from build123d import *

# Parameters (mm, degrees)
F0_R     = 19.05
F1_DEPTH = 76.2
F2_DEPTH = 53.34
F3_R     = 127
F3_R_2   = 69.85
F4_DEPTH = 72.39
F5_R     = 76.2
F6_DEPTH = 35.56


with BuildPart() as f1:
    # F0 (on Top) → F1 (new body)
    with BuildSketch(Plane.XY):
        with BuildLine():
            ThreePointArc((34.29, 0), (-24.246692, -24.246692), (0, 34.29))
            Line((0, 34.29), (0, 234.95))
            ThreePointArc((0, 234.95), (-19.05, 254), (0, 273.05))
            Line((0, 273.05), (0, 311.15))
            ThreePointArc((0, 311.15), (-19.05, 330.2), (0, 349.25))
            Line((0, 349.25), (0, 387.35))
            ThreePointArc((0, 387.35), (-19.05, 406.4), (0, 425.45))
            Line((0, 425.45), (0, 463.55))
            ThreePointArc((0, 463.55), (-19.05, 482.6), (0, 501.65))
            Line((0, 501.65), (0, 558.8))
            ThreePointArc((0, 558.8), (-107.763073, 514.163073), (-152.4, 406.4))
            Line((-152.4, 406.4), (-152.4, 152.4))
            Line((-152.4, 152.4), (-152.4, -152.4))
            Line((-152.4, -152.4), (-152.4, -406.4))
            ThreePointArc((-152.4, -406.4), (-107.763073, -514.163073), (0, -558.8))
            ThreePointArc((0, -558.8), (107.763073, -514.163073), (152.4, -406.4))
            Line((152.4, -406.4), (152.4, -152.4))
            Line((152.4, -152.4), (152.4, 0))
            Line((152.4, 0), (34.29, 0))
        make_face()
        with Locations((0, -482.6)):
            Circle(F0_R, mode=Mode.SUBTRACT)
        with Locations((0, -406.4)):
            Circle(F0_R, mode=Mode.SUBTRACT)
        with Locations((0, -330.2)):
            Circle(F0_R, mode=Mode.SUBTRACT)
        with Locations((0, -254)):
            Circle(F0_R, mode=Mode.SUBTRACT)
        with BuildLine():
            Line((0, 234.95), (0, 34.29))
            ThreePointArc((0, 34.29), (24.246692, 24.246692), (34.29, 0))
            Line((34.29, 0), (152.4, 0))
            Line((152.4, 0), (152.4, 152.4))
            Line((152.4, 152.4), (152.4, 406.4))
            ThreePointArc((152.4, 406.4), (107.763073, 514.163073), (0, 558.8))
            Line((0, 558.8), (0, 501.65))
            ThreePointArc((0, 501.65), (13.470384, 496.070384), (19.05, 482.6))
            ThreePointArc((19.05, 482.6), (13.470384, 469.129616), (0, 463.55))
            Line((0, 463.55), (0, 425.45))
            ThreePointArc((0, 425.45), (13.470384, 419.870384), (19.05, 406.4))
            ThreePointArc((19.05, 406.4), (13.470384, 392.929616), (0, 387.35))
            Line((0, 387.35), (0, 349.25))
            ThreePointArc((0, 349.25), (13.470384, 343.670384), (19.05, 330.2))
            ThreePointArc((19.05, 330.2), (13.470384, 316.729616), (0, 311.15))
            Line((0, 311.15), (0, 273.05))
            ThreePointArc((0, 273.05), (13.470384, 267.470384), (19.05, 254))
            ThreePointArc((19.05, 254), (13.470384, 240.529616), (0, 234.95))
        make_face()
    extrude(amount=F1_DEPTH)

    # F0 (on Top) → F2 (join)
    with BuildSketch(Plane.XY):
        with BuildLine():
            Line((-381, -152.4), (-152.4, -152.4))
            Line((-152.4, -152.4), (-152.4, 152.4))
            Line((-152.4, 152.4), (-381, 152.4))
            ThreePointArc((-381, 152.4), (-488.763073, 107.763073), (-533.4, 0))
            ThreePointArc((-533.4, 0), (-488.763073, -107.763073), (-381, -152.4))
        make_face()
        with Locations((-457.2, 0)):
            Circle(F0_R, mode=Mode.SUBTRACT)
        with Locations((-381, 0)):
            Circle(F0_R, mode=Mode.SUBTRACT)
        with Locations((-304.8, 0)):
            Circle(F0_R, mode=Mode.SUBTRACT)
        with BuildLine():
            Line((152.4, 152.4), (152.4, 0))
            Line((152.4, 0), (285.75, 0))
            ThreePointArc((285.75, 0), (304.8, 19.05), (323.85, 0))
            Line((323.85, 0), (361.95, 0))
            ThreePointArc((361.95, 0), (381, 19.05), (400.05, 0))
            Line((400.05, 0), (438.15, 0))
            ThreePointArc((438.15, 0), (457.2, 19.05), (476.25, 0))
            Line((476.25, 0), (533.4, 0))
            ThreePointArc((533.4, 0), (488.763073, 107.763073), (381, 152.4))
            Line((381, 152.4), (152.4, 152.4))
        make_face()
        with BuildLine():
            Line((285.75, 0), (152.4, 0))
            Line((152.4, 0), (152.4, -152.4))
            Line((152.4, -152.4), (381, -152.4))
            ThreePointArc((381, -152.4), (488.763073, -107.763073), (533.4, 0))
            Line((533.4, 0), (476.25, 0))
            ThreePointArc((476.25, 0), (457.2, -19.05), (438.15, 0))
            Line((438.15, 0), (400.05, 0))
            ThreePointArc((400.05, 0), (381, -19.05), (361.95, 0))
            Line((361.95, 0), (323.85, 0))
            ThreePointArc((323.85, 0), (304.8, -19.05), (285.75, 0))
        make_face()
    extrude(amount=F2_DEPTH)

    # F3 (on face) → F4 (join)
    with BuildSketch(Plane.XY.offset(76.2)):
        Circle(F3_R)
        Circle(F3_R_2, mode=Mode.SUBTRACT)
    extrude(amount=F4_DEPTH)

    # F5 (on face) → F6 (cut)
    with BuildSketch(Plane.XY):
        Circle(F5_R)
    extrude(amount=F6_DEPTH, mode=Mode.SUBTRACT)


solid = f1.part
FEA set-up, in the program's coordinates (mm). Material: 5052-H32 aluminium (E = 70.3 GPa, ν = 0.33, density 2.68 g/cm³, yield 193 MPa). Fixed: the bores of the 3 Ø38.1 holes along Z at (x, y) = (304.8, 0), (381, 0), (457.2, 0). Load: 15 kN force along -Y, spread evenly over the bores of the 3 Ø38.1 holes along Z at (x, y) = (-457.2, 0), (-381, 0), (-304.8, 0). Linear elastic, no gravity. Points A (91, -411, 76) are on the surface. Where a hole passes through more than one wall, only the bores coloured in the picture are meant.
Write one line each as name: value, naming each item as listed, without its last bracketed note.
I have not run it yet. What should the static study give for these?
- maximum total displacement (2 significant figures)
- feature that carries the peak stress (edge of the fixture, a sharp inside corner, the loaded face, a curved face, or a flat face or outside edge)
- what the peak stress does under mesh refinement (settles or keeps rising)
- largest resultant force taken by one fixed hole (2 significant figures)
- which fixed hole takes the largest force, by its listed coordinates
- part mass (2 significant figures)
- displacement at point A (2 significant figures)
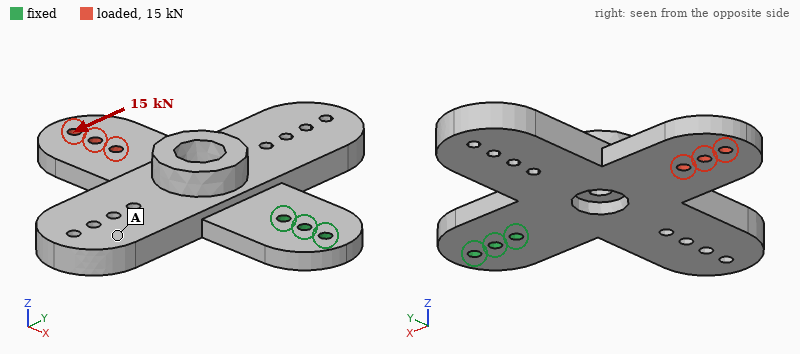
maximum total displacement: 0.42 mm
feature that carries the peak stress: edge of the fixture
what the peak stress does under mesh refinement: keeps rising
largest resultant force taken by one fixed hole: 69 kN
which fixed hole takes the largest force, by its listed coordinates: (304.8, 0)
part mass: 98 kg
displacement at point A: 0.22 mm
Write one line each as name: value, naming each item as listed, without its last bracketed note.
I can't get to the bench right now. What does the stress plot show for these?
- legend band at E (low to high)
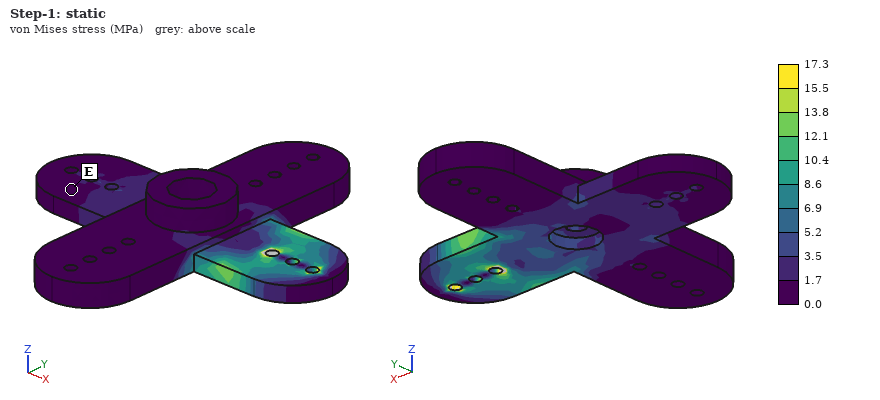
legend band at E: 0.0 to 1.7 MPa
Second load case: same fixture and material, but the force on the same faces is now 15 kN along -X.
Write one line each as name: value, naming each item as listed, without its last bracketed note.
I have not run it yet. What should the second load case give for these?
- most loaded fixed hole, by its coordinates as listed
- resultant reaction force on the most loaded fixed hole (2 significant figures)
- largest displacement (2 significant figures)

most loaded fixed hole, by its coordinates as listed: (304.8, 0)
resultant reaction force on the most loaded fixed hole: 9.5 kN
largest displacement: 36 µm
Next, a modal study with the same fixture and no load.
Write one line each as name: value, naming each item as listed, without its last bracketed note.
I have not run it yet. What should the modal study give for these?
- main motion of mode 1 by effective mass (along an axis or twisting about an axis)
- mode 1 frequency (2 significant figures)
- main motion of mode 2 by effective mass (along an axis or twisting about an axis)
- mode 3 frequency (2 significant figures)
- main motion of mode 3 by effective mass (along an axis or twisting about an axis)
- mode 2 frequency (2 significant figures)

main motion of mode 1 by effective mass: along Z
mode 1 frequency: 64 Hz
main motion of mode 2 by effective mass: twisting about X
mode 3 frequency: 170 Hz
main motion of mode 3 by effective mass: along Y
mode 2 frequency: 92 Hz
